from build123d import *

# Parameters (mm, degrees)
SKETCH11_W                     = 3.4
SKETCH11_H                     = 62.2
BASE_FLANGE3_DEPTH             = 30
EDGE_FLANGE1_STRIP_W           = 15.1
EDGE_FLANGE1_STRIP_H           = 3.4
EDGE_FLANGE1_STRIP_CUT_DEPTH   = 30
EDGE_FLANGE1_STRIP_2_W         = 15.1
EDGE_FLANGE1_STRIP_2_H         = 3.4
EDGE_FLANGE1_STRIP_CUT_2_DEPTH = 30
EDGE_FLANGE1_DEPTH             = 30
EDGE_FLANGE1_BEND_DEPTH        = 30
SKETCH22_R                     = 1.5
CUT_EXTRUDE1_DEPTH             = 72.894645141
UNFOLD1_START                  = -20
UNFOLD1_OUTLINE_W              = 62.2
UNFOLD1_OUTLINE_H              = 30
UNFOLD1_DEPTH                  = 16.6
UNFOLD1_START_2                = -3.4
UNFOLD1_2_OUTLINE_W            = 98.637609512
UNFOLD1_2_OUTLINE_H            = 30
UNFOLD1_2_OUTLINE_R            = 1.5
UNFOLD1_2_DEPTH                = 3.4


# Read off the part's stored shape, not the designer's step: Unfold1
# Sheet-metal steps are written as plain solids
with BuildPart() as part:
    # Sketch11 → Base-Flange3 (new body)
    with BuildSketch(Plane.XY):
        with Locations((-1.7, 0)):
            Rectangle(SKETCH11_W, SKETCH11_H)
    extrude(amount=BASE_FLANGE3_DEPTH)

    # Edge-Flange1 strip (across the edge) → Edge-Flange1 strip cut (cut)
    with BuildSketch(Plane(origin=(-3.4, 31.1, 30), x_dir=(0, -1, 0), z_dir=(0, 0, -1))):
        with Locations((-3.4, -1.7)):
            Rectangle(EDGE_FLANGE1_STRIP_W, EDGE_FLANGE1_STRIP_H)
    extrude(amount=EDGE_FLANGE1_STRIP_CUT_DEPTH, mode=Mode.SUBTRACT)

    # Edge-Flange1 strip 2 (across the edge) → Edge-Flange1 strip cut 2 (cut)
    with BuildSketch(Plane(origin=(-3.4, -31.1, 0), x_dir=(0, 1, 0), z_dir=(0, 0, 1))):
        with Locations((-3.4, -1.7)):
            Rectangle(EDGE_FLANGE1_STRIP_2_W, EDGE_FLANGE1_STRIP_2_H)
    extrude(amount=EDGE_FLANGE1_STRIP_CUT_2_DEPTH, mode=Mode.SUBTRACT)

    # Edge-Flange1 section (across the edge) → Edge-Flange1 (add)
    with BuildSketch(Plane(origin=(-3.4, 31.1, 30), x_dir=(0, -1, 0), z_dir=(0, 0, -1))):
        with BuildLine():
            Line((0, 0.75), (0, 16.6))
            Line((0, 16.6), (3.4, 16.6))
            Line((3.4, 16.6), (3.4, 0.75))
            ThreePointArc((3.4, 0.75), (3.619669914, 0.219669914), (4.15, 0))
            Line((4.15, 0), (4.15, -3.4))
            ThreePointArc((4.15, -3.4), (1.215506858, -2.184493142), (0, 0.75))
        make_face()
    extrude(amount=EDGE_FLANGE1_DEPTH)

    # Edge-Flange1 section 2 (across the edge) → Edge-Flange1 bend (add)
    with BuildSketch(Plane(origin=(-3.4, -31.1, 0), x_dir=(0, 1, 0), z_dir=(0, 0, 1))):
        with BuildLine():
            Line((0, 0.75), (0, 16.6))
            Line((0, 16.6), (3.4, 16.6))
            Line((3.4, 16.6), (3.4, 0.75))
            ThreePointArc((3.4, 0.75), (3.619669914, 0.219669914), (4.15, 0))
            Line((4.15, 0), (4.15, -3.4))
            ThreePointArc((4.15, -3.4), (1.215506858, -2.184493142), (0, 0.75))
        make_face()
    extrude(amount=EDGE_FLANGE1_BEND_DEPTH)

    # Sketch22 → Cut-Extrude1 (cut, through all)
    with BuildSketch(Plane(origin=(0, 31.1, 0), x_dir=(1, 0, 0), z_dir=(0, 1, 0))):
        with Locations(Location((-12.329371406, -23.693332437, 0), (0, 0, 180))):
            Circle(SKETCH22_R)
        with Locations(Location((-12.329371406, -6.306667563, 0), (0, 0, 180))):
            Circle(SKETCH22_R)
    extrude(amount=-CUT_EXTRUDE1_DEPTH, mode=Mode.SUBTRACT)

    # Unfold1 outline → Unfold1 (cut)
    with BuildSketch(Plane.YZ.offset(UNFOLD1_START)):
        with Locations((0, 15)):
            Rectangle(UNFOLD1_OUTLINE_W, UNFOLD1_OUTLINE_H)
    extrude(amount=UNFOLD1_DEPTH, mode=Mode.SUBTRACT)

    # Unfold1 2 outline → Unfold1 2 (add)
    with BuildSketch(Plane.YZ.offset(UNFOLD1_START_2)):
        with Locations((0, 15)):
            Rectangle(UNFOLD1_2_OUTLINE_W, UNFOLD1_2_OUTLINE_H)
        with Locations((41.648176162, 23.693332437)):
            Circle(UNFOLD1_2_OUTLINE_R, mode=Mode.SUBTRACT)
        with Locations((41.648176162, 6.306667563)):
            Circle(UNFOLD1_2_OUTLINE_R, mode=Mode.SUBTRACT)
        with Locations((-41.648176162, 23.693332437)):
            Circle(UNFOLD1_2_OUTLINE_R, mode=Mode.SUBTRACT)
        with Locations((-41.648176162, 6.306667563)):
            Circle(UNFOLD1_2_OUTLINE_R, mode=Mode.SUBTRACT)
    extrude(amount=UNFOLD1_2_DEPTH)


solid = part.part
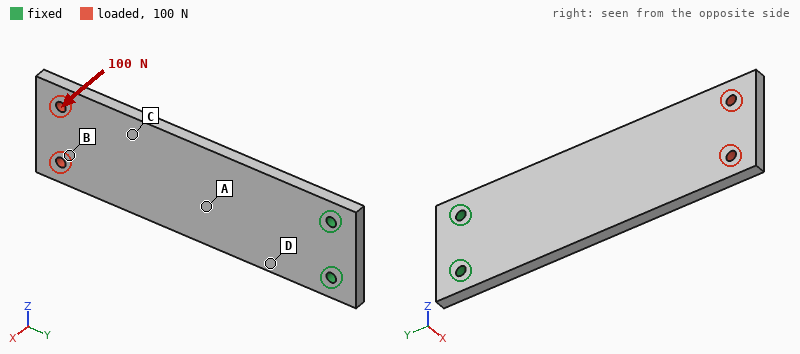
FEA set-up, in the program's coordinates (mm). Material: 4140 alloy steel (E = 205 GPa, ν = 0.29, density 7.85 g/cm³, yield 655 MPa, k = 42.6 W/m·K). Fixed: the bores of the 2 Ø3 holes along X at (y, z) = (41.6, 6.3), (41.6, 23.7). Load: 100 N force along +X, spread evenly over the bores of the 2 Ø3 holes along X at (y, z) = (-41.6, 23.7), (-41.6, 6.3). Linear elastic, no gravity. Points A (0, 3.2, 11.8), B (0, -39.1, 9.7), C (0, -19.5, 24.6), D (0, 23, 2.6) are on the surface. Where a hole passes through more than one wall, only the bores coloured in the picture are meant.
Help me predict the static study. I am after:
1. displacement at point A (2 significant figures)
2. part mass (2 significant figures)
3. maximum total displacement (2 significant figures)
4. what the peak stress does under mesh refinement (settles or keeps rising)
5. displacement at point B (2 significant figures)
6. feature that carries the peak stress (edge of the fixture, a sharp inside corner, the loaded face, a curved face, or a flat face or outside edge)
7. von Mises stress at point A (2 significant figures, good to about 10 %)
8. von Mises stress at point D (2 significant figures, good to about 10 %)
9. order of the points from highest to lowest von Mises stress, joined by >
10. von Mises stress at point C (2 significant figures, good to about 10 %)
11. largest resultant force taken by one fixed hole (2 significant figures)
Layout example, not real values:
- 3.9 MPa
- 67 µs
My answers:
- 0.26 mm
- 78 g
- 1.1 mm
- keeps rising
- 0.91 mm
- edge of the fixture
- 77 MPa
- 110 MPa
- D > A > C > B
- 39 MPa
- 50 N
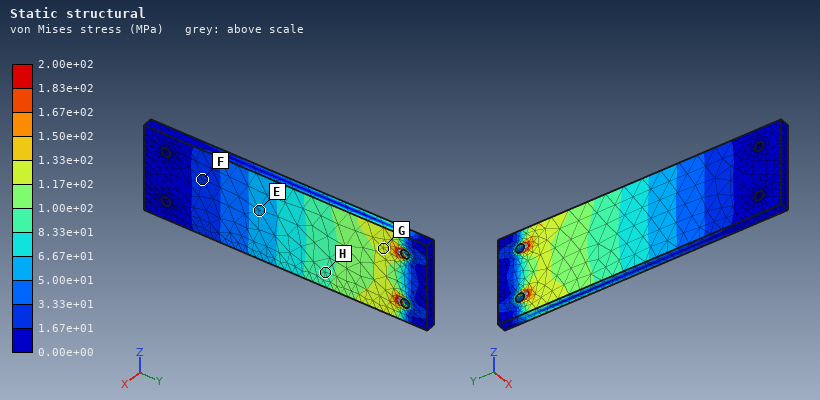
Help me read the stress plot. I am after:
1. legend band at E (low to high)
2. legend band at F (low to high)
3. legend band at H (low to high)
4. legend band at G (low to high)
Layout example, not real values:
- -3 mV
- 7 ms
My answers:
- 5.00e+01 to 6.67e+01 MPa
- 1.67e+01 to 3.33e+01 MPa
- 8.33e+01 to 1.00e+02 MPa
- 1.17e+02 to 1.33e+02 MPa
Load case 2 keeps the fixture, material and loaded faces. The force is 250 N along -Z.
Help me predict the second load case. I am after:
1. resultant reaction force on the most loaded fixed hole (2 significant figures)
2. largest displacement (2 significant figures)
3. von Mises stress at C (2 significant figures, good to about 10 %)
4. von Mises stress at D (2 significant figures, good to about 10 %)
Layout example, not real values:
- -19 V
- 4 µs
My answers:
- 1.1 kN
- 43 µm
- 7.9 MPa
- 26 MPa
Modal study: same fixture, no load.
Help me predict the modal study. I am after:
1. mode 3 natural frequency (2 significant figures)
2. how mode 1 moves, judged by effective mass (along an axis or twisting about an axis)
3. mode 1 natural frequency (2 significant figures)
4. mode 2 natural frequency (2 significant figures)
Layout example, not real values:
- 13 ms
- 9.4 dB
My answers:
- 2100 Hz
- along X
- 340 Hz
- 2100 Hz
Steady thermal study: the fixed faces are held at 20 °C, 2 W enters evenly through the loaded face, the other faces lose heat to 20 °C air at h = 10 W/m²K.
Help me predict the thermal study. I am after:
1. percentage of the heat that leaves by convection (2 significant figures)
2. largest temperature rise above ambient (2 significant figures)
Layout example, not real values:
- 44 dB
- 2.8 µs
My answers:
- 42 %
- 28 K
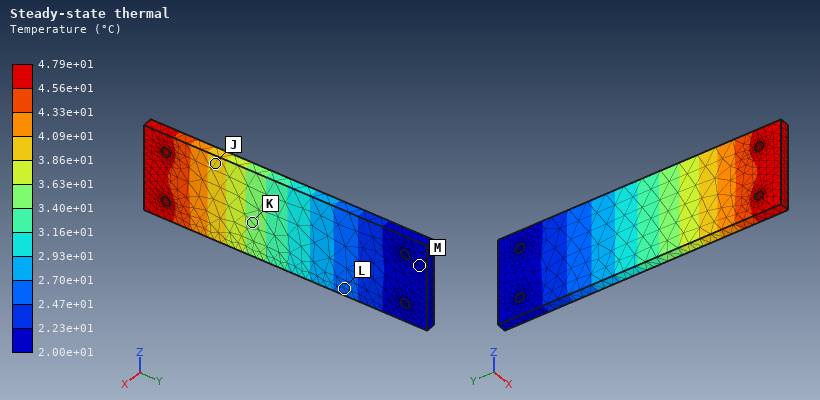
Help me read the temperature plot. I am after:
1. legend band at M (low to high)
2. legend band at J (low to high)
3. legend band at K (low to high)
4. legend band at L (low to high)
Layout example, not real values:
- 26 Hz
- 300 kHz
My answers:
- 2.00e+01 to 2.23e+01 °C
- 3.86e+01 to 4.09e+01 °C
- 3.40e+01 to 3.63e+01 °C
- 2.47e+01 to 2.70e+01 °C
